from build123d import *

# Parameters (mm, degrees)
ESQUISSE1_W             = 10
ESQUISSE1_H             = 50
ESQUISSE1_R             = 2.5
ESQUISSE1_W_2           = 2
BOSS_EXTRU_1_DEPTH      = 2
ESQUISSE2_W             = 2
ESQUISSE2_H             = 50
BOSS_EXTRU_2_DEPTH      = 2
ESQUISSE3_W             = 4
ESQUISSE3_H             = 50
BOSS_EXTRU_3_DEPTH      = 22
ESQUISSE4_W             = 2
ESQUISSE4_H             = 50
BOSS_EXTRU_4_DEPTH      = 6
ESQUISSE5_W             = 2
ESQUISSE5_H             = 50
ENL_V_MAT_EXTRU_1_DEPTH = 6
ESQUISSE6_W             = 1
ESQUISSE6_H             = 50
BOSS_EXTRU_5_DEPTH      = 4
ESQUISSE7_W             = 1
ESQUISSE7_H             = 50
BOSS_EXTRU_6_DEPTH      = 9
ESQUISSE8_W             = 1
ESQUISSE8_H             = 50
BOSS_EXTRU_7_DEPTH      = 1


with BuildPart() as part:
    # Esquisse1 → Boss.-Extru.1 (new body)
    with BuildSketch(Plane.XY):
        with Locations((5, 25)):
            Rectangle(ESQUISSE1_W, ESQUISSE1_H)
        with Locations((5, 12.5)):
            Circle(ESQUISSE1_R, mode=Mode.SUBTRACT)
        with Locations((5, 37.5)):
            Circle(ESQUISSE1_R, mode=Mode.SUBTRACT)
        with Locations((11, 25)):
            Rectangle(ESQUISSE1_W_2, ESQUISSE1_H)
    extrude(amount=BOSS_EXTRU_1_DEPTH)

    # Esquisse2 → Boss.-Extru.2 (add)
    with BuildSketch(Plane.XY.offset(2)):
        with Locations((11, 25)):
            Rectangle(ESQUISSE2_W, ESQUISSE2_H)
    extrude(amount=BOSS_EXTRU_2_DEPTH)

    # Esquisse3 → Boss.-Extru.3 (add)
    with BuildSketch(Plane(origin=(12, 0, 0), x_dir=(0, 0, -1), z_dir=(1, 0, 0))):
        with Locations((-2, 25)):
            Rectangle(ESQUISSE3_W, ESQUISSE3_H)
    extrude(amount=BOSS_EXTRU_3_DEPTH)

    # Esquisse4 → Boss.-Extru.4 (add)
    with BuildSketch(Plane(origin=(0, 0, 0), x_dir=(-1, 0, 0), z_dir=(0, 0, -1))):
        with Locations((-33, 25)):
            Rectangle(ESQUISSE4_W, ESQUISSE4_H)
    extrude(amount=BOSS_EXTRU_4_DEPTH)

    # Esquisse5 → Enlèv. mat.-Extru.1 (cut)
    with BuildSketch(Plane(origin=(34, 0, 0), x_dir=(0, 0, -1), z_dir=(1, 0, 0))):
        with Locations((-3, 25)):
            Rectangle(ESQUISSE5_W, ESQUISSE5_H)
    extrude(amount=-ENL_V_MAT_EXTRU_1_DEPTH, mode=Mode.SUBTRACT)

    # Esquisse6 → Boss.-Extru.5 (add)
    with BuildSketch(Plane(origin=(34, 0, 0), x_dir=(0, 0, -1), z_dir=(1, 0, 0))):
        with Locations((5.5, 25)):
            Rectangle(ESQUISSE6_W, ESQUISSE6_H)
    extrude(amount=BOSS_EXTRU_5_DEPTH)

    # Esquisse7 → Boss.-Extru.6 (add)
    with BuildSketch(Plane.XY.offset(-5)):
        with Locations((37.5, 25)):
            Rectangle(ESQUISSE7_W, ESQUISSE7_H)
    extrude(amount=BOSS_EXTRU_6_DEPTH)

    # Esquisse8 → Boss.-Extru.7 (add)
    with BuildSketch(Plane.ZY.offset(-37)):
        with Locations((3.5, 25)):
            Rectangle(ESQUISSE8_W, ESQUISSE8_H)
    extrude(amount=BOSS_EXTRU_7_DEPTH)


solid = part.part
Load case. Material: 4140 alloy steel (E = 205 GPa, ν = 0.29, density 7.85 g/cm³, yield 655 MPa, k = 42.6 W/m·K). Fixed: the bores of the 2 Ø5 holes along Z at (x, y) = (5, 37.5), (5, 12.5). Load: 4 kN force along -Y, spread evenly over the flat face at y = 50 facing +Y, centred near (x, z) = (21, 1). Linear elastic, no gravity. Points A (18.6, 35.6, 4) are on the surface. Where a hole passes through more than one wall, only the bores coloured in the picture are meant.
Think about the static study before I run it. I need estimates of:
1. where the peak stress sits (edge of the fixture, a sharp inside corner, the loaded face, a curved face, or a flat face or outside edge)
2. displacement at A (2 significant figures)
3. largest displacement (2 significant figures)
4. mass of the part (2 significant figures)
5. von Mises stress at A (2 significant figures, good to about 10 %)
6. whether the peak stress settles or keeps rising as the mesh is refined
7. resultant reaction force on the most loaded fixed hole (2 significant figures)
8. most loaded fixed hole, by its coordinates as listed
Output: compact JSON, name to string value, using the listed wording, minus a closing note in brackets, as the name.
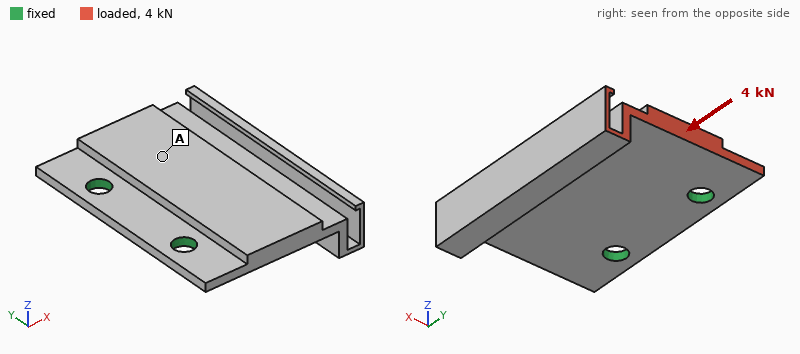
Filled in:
{"where the peak stress sits": "edge of the fixture", "displacement at A": "13 µm", "largest displacement": "51 µm", "mass of the part": "50 g", "von Mises stress at A": "32 MPa", "whether the peak stress settles or keeps rising as the mesh is refined": "keeps rising", "resultant reaction force on the most loaded fixed hole": "3.2 kN", "most loaded fixed hole, by its coordinates as listed": "(5, 37.5)"}
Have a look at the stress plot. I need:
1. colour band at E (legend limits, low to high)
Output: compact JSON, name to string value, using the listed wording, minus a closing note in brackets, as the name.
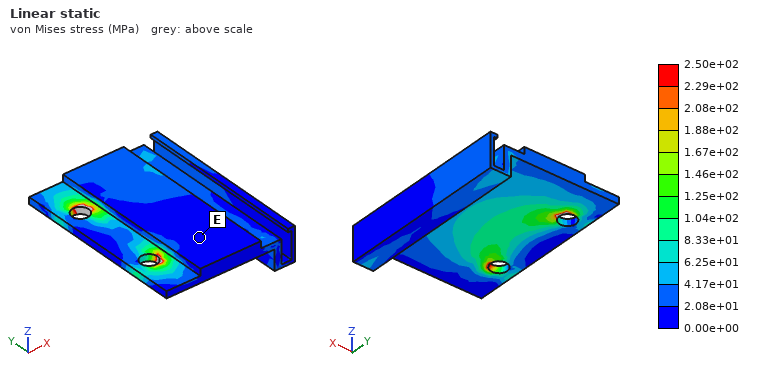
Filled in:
{"colour band at E": "0.00e+00 to 2.08e+01 MPa"}
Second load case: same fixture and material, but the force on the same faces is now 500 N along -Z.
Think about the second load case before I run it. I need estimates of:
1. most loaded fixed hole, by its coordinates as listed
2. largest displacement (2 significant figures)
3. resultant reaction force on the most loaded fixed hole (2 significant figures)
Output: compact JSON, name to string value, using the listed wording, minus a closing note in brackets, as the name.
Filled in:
{"most loaded fixed hole, by its coordinates as listed": "(5, 37.5)", "largest displacement": "0.27 mm", "resultant reaction force on the most loaded fixed hole": "660 N"}
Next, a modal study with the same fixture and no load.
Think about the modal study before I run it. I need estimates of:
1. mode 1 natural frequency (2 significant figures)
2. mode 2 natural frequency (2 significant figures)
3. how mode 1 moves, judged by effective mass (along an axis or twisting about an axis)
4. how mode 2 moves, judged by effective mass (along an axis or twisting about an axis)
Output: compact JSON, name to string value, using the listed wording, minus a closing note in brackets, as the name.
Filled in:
{"mode 1 natural frequency": "1400 Hz", "mode 2 natural frequency": "3300 Hz", "how mode 1 moves, judged by effective mass": "along Z", "how mode 2 moves, judged by effective mass": "twisting about X"}
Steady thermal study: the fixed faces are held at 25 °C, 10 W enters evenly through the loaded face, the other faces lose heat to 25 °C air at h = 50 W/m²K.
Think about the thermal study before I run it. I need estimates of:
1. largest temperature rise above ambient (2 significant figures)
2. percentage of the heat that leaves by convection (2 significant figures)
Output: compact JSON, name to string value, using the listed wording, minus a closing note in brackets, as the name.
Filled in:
{"largest temperature rise above ambient": "40 K", "percentage of the heat that leaves by convection": "39 %"}
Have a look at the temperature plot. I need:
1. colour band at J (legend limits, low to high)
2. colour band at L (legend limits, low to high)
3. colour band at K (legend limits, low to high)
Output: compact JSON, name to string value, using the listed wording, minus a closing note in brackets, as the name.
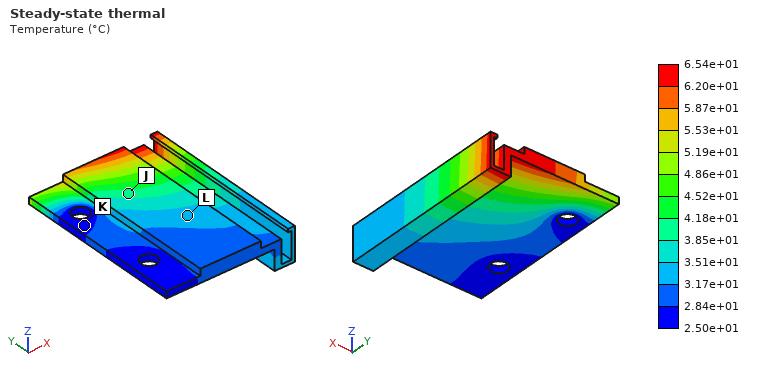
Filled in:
{"colour band at J": "3.85e+01 to 4.18e+01 °C", "colour band at L": "3.17e+01 to 3.51e+01 °C", "colour band at K": "2.50e+01 to 2.84e+01 °C"}
